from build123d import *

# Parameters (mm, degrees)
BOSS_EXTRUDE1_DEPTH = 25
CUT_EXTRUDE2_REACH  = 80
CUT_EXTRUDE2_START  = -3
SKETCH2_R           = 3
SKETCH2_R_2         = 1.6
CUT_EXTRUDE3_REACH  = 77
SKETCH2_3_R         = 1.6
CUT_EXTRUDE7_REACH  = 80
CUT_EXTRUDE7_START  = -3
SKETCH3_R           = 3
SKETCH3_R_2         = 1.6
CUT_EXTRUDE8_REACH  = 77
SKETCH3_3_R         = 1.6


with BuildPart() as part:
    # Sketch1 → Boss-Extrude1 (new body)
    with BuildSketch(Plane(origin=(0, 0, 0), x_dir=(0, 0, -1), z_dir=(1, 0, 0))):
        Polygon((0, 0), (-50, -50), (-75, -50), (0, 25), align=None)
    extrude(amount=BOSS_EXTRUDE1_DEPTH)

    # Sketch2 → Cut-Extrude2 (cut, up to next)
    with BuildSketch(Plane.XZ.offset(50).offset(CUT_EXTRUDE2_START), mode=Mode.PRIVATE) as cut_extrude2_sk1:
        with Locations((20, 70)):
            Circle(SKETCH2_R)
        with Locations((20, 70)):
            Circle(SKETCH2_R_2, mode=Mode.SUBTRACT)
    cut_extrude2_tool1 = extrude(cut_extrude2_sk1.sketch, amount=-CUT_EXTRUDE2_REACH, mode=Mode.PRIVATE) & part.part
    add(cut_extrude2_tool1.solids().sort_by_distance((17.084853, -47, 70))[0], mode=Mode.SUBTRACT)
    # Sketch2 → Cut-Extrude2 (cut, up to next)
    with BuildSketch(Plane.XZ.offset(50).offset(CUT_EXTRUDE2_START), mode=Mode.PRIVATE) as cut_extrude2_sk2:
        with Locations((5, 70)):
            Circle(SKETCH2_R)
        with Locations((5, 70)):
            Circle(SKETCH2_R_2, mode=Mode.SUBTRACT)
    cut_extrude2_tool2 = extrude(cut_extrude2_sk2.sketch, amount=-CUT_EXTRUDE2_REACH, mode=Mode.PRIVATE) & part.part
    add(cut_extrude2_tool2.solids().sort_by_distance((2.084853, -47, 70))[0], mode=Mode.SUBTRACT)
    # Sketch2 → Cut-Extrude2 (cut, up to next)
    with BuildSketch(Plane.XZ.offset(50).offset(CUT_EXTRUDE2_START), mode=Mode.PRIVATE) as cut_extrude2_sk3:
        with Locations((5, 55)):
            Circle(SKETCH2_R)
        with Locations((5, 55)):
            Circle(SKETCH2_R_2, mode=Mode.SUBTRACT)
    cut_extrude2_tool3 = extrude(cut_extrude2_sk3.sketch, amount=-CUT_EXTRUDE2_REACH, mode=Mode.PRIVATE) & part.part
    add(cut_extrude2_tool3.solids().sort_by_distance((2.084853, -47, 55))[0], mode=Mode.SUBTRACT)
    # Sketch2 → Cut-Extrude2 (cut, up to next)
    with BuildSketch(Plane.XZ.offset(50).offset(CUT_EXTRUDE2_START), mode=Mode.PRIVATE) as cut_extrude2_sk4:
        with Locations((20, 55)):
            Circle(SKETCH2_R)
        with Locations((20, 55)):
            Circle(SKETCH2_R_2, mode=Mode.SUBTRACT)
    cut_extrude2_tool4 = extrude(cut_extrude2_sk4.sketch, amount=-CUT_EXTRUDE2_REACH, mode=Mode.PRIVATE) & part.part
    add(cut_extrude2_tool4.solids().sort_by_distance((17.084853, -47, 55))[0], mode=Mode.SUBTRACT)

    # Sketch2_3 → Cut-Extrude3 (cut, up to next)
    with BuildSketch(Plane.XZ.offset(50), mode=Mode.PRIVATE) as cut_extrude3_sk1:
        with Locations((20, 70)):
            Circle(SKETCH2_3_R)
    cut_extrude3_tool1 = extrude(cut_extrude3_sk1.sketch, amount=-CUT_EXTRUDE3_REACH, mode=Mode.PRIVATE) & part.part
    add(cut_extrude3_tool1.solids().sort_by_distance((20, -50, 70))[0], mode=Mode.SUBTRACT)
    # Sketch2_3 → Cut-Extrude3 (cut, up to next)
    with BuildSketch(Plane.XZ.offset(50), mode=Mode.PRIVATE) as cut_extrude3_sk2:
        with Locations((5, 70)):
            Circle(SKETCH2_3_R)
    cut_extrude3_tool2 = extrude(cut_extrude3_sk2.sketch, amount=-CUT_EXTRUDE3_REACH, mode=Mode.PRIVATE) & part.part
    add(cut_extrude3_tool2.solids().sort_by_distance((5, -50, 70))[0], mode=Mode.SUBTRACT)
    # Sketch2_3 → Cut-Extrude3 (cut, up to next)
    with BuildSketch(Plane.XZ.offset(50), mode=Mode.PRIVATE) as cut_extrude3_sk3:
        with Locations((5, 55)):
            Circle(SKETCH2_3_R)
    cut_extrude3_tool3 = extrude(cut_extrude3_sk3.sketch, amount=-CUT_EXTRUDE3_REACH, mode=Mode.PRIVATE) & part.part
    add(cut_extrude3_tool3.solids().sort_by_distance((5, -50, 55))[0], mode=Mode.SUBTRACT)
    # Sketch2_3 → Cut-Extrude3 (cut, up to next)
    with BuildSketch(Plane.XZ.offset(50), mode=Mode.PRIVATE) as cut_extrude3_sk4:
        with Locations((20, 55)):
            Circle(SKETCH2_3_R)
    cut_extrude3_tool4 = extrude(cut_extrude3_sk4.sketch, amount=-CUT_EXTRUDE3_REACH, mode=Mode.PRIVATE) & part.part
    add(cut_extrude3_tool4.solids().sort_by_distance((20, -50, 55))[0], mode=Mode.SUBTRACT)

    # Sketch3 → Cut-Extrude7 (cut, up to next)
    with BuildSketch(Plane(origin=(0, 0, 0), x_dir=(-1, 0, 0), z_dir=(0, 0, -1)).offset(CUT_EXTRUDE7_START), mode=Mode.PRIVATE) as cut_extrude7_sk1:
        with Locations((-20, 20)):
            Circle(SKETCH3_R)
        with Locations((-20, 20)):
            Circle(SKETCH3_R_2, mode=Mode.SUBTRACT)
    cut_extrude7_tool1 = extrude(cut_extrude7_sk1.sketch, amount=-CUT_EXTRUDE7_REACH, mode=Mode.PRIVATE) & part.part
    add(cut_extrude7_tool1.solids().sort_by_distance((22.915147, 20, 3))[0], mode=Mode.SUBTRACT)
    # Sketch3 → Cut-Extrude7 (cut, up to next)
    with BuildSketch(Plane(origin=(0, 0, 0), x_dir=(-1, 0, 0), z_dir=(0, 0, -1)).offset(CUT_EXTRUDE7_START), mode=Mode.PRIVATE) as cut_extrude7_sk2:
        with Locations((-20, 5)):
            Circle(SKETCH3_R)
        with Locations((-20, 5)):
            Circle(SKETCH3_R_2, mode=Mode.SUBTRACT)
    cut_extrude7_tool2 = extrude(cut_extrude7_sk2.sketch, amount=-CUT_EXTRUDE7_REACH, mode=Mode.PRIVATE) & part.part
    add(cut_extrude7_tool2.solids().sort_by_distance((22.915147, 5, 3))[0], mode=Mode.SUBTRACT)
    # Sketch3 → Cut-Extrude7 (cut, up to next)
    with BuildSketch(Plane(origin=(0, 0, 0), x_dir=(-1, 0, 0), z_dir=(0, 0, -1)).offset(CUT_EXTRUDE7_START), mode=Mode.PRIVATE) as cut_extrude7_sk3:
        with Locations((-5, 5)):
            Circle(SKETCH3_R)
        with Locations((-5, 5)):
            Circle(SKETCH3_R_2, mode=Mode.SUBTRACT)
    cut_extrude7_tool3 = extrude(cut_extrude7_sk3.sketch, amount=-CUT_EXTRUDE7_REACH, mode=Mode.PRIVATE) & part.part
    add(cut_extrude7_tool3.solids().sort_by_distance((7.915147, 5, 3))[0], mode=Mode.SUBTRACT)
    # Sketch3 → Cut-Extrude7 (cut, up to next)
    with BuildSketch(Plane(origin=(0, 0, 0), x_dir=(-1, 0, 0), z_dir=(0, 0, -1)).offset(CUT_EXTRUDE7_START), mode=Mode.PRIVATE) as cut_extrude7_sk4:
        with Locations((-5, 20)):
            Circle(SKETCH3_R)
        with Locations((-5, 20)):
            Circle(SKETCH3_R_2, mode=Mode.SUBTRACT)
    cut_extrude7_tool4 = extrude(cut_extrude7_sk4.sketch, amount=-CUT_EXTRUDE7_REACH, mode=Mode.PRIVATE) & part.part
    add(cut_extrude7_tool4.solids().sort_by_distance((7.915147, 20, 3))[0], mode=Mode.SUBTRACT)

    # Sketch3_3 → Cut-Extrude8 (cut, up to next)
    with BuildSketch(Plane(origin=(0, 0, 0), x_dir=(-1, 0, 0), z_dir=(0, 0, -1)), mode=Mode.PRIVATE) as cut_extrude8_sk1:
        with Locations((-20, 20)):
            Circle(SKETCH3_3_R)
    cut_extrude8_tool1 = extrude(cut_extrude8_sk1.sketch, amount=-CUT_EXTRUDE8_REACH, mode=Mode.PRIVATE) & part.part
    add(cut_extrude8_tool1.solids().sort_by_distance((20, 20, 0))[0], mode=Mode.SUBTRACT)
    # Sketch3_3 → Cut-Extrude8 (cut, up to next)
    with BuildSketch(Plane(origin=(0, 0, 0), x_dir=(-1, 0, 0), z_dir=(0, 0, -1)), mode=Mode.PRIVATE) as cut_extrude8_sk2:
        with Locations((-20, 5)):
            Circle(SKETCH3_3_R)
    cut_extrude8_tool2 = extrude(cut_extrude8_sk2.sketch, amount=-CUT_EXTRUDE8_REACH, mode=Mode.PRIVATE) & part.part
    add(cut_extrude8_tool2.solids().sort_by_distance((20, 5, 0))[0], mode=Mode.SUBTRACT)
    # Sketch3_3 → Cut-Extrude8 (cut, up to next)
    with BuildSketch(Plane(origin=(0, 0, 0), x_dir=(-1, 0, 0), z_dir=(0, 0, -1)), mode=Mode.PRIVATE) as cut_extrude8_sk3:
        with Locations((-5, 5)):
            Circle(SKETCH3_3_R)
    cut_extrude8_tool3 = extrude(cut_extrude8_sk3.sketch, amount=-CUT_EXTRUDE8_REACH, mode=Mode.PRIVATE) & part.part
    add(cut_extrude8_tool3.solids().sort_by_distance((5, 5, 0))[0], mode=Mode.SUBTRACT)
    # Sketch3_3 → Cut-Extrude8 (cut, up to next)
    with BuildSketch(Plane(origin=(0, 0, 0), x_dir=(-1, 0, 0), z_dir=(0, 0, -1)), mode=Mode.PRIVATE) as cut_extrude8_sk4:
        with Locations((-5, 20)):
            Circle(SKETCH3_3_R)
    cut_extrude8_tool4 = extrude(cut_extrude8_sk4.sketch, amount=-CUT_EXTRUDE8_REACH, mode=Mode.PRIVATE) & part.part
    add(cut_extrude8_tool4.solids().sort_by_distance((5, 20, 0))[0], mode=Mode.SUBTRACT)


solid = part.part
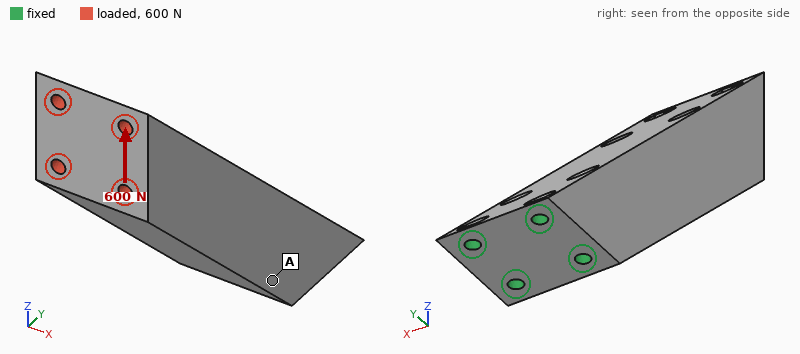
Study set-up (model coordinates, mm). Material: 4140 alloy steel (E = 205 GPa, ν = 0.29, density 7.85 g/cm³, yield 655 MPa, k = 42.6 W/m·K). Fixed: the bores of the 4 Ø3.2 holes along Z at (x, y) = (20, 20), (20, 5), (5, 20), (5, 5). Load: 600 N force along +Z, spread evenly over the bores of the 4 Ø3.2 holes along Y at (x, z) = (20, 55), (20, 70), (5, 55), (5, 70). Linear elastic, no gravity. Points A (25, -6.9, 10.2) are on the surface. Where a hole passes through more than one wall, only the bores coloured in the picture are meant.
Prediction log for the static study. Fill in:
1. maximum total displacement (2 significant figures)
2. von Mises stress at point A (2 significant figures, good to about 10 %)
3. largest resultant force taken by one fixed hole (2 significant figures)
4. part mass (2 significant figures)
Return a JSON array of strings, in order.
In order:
["69 µm", "18 MPa", "1.4 kN", "290 g"]
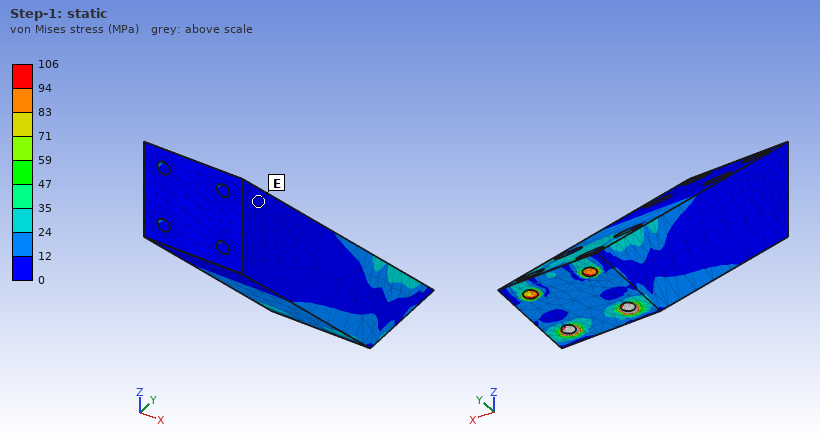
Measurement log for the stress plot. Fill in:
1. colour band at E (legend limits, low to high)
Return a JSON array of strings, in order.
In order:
["0 to 12 MPa"]
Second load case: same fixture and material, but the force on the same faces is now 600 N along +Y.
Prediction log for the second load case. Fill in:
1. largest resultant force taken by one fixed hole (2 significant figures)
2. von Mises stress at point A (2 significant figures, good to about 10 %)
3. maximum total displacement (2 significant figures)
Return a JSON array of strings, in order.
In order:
["1.3 kN", "16 MPa", "74 µm"]
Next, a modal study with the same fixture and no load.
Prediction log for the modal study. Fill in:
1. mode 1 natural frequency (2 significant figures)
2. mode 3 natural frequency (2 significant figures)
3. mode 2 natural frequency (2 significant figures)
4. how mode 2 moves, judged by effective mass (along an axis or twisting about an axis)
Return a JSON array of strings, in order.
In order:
["1500 Hz", "7600 Hz", "2100 Hz", "along X"]
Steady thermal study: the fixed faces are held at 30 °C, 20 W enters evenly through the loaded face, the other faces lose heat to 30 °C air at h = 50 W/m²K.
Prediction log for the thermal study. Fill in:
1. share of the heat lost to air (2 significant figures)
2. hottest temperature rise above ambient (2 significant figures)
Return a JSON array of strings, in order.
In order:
["62 %", "72 K"]
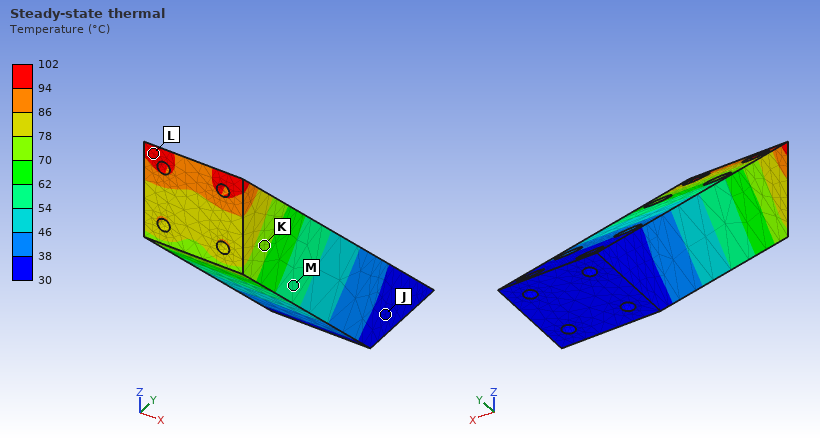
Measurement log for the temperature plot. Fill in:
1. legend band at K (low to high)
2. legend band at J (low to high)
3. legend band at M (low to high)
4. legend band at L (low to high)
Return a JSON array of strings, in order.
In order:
["70 to 78 °C", "30 to 38 °C", "54 to 62 °C", "94 to 102 °C"]
